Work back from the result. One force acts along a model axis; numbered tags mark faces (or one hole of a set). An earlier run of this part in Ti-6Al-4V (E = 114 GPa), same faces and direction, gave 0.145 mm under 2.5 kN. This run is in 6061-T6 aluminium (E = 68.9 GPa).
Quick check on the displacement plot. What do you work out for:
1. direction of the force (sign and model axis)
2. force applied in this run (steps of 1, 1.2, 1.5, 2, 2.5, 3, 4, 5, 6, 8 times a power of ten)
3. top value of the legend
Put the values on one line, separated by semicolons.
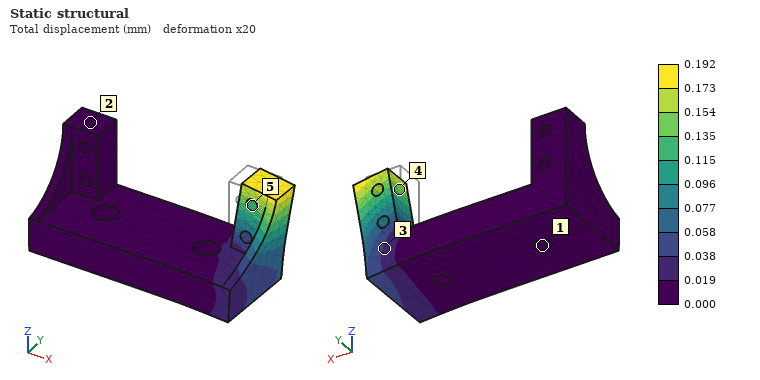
+X; 2 kN; 0.192 mm
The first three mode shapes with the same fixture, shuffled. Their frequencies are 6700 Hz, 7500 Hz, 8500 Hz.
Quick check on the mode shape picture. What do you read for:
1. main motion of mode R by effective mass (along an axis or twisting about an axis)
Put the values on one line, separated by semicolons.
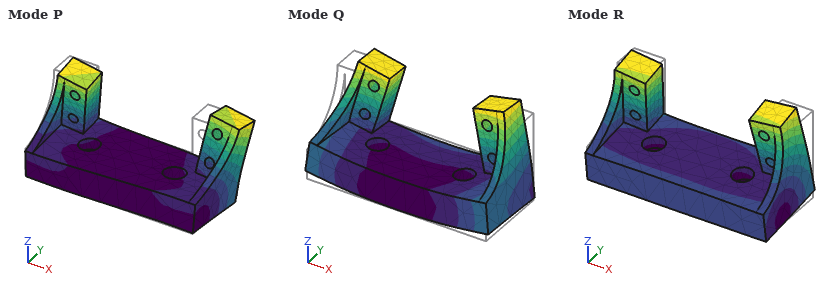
along Y
